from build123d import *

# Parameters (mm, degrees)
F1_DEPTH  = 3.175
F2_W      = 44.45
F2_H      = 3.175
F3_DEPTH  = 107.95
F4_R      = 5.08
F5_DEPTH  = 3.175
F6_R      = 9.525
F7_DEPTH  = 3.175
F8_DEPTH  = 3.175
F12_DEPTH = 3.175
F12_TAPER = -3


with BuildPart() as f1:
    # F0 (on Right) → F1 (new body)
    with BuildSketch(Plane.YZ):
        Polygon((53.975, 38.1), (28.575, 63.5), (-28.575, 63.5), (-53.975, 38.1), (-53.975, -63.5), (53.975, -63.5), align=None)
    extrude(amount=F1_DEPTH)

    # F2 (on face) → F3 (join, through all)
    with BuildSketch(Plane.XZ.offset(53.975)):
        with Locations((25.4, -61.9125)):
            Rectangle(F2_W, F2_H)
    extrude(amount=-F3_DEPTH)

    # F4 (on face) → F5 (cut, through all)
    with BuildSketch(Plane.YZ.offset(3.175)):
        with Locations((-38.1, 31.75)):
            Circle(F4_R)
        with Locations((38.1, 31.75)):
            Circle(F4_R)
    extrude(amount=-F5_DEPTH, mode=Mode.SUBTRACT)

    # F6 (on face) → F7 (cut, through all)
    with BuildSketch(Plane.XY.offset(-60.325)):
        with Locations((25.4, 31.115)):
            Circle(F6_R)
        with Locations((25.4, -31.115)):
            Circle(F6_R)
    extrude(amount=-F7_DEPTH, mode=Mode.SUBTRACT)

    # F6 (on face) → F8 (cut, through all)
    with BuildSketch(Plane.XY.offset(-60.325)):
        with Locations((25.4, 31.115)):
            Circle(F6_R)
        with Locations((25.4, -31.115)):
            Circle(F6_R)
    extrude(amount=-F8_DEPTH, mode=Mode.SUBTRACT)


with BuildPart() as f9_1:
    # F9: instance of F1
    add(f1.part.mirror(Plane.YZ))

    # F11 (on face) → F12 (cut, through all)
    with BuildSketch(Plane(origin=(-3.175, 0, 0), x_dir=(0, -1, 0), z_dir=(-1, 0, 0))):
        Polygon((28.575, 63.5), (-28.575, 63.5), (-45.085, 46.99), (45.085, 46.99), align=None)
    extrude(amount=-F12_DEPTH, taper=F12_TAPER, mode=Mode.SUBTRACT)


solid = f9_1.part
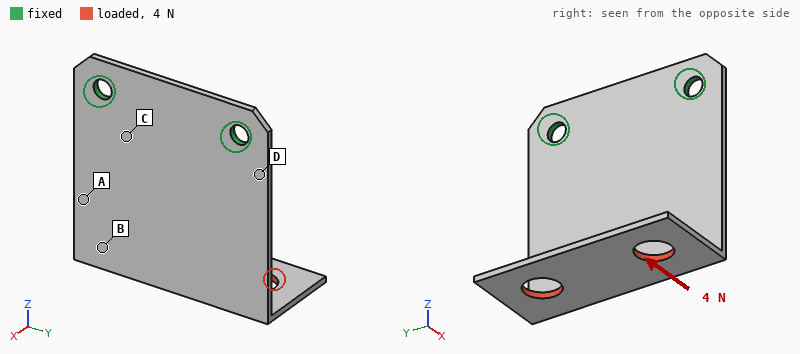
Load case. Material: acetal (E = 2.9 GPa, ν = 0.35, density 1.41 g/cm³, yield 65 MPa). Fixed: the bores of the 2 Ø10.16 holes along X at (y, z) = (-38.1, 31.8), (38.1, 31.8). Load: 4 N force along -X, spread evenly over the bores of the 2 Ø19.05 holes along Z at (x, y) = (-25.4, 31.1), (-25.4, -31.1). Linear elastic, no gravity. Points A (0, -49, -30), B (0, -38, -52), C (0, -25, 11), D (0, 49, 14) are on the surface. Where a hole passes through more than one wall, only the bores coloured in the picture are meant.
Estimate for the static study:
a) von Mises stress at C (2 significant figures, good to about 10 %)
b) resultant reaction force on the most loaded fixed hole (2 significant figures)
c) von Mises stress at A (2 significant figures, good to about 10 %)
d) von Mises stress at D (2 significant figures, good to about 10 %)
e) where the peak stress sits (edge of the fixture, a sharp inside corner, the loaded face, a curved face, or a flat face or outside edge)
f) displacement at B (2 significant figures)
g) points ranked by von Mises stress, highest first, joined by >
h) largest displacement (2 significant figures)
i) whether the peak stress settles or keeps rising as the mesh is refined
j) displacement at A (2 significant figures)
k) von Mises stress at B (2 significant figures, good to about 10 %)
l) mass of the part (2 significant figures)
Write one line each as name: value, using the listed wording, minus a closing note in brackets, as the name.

von Mises stress at C: 1.4 MPa
resultant reaction force on the most loaded fixed hole: 2.0 N
von Mises stress at A: 0.77 MPa
von Mises stress at D: 2.0 MPa
where the peak stress sits: edge of the fixture
displacement at B: 1.1 mm
points ranked by von Mises stress, highest first, joined by >: D > C > A > B
largest displacement: 1.6 mm
whether the peak stress settles or keeps rising as the mesh is refined: keeps rising
displacement at A: 0.62 mm
von Mises stress at B: 0.28 MPa
mass of the part: 71 g
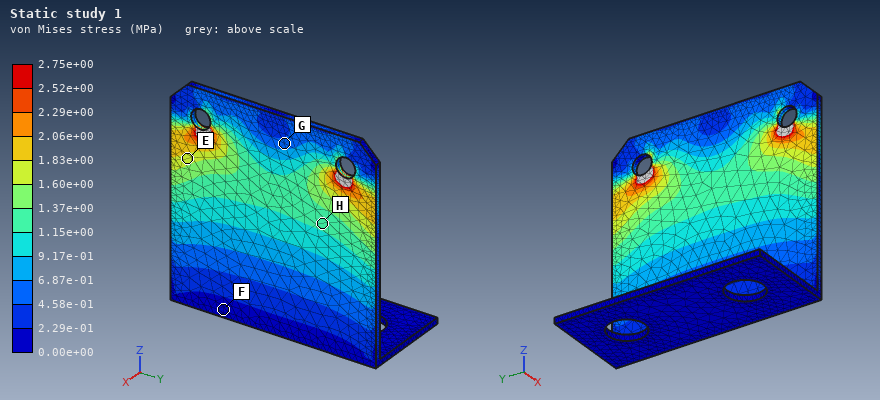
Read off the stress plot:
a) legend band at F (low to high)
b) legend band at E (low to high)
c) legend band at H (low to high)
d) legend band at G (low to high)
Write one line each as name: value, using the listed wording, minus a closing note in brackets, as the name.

legend band at F: 0.00e+00 to 2.29e-01 MPa
legend band at E: 1.60e+00 to 1.83e+00 MPa
legend band at H: 1.15e+00 to 1.37e+00 MPa
legend band at G: 4.58e-01 to 6.87e-01 MPa
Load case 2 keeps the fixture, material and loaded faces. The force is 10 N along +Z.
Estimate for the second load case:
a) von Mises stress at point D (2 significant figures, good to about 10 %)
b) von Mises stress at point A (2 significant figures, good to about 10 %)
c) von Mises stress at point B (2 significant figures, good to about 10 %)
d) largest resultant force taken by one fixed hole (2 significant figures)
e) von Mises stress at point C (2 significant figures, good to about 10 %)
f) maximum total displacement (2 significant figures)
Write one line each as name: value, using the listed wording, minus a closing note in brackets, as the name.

von Mises stress at point D: 1.5 MPa
von Mises stress at point A: 1.3 MPa
von Mises stress at point B: 1.1 MPa
largest resultant force taken by one fixed hole: 5.1 N
von Mises stress at point C: 1.2 MPa
maximum total displacement: 1.8 mm
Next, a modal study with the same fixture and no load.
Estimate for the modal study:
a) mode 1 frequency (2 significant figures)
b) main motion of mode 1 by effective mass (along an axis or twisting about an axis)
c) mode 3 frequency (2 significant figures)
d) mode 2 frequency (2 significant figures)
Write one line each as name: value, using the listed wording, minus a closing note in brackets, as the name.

mode 1 frequency: 49 Hz
main motion of mode 1 by effective mass: along X
mode 3 frequency: 200 Hz
mode 2 frequency: 110 Hz
